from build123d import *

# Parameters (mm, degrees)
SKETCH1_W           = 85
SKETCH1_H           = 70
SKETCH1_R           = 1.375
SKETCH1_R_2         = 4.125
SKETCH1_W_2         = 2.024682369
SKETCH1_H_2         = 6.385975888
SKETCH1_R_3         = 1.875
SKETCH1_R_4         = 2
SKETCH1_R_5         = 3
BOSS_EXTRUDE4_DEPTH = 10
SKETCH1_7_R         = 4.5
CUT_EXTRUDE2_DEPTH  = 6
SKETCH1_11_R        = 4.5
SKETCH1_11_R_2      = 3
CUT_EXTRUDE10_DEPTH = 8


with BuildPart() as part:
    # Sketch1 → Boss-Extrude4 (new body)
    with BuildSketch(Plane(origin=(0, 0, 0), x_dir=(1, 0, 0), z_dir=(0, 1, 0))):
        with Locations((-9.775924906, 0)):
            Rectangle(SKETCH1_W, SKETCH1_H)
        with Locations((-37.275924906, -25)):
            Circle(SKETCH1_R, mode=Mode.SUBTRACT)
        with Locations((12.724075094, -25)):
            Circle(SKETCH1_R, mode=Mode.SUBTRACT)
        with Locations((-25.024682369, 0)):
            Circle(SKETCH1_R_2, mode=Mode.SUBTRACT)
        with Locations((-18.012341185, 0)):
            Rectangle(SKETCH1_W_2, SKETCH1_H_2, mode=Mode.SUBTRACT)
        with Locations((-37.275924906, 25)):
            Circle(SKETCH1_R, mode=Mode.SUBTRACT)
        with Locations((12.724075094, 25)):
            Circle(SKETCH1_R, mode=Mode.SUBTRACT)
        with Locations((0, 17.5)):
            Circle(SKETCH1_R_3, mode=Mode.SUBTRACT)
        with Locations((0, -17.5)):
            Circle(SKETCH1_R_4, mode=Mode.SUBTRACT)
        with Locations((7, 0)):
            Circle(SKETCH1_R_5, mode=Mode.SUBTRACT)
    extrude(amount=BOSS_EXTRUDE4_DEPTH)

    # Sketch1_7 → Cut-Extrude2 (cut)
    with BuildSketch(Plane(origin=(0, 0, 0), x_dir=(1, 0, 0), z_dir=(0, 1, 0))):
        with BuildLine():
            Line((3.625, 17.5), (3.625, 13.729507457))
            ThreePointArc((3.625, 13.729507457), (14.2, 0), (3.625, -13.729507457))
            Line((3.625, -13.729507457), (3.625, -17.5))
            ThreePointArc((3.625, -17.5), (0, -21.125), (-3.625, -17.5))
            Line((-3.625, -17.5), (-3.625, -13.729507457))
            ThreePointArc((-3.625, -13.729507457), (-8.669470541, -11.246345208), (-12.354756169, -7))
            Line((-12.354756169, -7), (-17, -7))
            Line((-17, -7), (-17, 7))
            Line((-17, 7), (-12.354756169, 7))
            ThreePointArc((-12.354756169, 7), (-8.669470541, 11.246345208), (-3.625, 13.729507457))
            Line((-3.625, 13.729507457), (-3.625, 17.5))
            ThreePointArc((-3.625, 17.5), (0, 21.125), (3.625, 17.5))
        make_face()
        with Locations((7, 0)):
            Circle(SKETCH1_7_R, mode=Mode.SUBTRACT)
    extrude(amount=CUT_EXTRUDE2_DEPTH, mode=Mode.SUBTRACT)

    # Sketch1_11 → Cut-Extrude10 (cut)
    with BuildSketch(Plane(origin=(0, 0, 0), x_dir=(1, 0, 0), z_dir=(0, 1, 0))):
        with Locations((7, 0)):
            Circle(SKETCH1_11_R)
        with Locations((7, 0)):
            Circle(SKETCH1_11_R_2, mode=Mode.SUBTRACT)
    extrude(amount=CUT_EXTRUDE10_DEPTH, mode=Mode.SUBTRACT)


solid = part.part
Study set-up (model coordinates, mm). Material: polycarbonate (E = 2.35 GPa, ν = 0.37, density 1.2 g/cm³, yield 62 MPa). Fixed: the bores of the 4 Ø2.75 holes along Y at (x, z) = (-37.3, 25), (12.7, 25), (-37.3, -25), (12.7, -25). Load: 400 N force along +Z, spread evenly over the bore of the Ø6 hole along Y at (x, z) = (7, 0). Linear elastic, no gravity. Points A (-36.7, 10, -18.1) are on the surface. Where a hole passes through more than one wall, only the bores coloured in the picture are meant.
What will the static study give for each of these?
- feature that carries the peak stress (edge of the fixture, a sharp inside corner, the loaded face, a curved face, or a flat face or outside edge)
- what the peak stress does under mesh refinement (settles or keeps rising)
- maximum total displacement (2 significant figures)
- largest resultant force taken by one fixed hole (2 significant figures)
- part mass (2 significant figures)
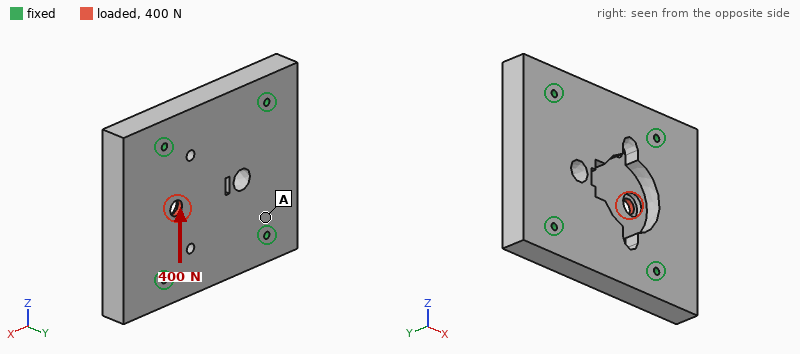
a sharp inside corner
keeps rising
39 µm
170 N
64 g
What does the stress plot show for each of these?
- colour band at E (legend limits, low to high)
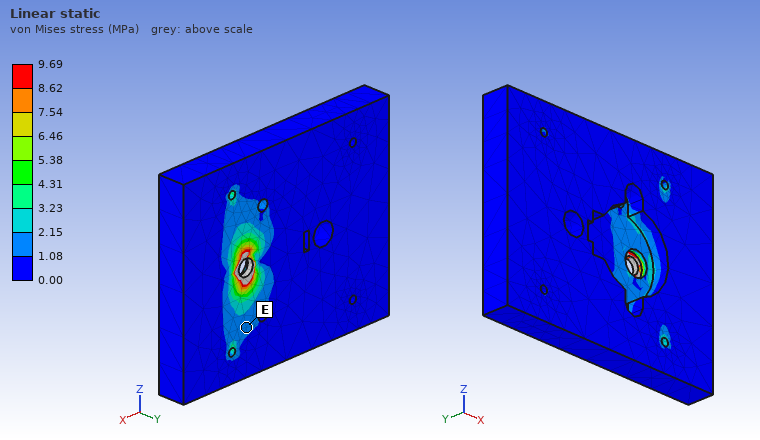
1.08 to 2.15 MPa
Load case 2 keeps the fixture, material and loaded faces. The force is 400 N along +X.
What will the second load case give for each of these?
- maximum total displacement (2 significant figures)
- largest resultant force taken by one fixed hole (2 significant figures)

53 µm
120 N
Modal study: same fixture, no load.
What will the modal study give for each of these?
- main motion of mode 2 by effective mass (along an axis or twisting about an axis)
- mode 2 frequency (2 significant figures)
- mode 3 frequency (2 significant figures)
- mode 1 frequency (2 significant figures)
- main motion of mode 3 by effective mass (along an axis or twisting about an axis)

along Y
3000 Hz
3600 Hz
2700 Hz
twisting about Z
